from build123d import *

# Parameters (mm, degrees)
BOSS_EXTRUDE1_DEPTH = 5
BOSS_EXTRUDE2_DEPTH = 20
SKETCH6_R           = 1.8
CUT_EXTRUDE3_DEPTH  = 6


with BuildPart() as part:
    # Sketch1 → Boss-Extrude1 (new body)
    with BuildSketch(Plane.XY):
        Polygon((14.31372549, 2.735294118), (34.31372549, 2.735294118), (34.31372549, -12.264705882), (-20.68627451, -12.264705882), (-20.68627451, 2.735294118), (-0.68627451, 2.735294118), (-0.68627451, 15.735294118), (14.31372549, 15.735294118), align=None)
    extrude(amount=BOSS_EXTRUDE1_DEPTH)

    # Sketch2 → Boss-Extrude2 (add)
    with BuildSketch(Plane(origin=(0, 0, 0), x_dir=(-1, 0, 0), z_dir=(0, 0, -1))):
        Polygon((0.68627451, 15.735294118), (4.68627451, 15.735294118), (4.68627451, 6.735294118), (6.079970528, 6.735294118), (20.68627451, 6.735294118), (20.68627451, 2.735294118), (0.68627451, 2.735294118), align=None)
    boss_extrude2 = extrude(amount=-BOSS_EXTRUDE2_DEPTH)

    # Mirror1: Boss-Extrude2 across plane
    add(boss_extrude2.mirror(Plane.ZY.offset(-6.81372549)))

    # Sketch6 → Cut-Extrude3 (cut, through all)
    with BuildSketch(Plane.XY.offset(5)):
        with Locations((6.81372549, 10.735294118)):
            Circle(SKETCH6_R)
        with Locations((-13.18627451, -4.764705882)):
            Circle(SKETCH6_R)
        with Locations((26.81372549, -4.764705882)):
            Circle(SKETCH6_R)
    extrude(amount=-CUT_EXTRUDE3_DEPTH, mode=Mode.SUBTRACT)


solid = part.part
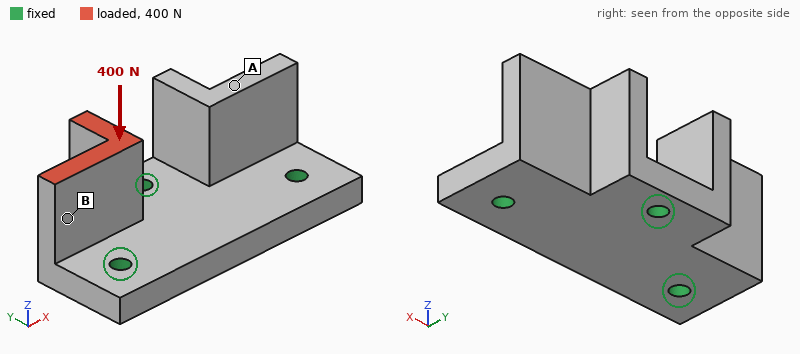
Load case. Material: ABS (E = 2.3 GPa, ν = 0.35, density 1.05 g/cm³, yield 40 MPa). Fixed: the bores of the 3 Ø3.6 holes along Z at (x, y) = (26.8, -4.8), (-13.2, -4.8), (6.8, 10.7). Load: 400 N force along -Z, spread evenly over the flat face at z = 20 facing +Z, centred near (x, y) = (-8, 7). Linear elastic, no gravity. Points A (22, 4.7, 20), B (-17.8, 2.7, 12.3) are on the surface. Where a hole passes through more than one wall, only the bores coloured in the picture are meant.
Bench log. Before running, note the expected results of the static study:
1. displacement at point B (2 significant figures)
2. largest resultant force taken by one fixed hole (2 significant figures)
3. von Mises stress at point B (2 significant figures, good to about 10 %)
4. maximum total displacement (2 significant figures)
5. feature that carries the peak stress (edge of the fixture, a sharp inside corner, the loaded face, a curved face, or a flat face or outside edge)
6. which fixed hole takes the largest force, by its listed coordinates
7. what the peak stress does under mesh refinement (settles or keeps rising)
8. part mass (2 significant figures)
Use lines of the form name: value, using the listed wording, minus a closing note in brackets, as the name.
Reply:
displacement at point B: 0.23 mm
largest resultant force taken by one fixed hole: 230 N
von Mises stress at point B: 5.9 MPa
maximum total displacement: 0.36 mm
feature that carries the peak stress: edge of the fixture
which fixed hole takes the largest force, by its listed coordinates: (-13.2, -4.8)
what the peak stress does under mesh refinement: keeps rising
part mass: 10 g
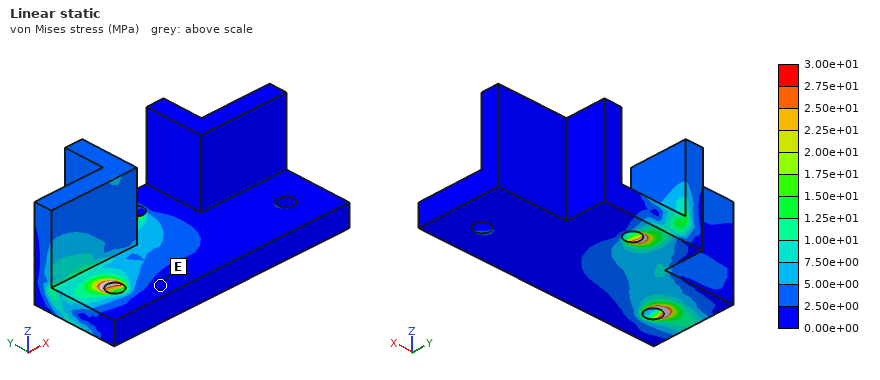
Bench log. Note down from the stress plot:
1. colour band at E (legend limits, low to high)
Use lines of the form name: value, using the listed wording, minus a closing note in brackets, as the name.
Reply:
colour band at E: 0.00e+00 to 2.50e+00 MPa
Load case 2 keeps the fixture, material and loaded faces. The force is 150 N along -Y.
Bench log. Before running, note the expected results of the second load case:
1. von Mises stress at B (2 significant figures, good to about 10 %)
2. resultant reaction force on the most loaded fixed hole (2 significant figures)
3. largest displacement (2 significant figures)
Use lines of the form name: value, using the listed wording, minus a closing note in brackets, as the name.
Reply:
von Mises stress at B: 8.8 MPa
resultant reaction force on the most loaded fixed hole: 120 N
largest displacement: 0.67 mm
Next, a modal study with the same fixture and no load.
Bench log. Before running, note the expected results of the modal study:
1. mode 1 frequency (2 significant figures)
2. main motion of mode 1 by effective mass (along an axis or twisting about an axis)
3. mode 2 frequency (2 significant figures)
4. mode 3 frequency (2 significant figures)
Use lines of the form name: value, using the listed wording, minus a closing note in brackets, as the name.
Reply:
mode 1 frequency: 2800 Hz
main motion of mode 1 by effective mass: along Y
mode 2 frequency: 3100 Hz
mode 3 frequency: 4800 Hz
